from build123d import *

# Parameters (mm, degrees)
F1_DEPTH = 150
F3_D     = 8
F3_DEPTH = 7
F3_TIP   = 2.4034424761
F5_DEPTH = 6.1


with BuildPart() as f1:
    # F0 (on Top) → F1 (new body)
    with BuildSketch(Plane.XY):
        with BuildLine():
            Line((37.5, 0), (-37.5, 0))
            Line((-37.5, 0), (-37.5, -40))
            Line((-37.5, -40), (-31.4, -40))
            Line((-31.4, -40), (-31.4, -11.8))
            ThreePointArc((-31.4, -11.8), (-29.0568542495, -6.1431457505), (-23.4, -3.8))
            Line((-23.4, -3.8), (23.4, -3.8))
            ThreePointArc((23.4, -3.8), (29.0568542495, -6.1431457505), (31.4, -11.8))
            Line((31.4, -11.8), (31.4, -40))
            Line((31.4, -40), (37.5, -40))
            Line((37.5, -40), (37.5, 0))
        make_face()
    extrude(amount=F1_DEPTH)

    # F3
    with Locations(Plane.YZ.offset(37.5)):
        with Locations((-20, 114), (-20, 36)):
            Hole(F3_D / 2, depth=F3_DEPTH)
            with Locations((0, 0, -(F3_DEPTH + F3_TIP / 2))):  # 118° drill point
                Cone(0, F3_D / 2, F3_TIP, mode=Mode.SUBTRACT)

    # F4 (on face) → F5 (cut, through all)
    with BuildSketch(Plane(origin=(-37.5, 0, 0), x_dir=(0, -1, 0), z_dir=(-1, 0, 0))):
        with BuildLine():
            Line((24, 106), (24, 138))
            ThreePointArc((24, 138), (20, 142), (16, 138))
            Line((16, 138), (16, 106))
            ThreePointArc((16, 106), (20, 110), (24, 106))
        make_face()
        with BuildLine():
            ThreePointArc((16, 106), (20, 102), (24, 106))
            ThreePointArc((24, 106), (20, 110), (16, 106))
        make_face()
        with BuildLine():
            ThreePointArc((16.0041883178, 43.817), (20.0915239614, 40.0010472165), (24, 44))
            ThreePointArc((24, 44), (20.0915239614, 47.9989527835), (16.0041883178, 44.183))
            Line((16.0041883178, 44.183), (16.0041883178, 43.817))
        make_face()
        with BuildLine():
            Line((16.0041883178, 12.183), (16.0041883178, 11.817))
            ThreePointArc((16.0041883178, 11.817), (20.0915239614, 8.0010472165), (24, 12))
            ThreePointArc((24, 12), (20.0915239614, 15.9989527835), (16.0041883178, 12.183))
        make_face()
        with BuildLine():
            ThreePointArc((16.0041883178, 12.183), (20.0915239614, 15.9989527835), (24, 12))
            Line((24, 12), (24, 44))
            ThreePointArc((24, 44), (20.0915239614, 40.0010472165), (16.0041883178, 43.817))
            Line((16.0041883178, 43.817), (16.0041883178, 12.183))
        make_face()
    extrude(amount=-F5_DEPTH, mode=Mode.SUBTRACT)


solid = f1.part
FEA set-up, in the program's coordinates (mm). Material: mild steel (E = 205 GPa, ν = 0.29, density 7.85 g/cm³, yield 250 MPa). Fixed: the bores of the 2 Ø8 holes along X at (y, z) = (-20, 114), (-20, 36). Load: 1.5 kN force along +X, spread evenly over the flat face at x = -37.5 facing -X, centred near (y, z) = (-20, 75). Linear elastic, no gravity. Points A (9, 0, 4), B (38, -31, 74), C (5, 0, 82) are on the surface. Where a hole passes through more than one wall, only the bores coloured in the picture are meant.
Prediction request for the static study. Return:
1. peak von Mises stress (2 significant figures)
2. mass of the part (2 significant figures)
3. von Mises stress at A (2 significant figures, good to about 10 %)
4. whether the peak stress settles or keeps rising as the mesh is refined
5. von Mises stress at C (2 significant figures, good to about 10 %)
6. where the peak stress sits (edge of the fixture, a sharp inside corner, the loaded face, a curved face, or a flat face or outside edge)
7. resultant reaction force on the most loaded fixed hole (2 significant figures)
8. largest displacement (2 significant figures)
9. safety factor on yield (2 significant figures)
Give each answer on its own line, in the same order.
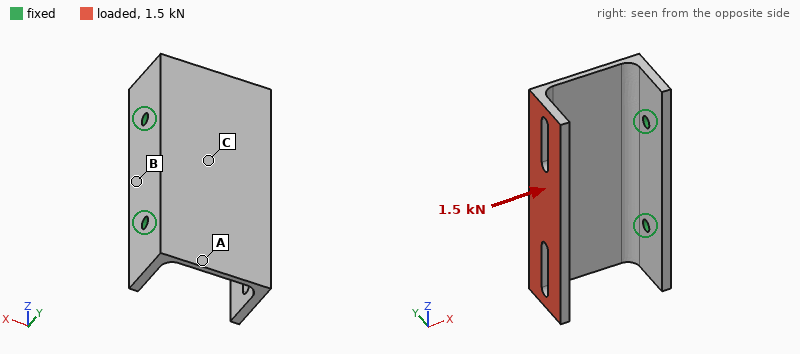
79 MPa
850 g
74 MPa
settles
65 MPa
a curved face
750 N
0.58 mm
3.2
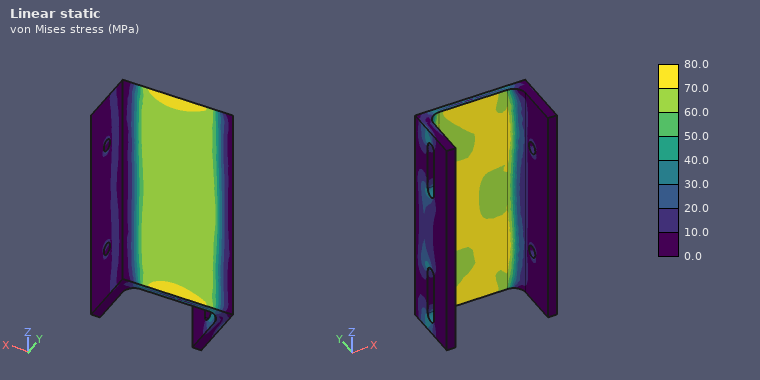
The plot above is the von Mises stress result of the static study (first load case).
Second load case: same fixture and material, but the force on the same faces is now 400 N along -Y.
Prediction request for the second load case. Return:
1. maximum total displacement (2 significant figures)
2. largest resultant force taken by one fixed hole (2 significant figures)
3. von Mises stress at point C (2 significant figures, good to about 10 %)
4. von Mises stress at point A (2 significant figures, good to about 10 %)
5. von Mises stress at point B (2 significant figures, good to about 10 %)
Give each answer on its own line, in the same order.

0.39 mm
200 N
42 MPa
51 MPa
7.8 MPa
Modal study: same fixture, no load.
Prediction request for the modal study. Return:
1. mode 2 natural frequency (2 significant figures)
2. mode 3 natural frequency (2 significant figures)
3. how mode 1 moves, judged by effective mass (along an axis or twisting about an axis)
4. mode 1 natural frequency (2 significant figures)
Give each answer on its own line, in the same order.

610 Hz
1200 Hz
along Y
310 Hz
